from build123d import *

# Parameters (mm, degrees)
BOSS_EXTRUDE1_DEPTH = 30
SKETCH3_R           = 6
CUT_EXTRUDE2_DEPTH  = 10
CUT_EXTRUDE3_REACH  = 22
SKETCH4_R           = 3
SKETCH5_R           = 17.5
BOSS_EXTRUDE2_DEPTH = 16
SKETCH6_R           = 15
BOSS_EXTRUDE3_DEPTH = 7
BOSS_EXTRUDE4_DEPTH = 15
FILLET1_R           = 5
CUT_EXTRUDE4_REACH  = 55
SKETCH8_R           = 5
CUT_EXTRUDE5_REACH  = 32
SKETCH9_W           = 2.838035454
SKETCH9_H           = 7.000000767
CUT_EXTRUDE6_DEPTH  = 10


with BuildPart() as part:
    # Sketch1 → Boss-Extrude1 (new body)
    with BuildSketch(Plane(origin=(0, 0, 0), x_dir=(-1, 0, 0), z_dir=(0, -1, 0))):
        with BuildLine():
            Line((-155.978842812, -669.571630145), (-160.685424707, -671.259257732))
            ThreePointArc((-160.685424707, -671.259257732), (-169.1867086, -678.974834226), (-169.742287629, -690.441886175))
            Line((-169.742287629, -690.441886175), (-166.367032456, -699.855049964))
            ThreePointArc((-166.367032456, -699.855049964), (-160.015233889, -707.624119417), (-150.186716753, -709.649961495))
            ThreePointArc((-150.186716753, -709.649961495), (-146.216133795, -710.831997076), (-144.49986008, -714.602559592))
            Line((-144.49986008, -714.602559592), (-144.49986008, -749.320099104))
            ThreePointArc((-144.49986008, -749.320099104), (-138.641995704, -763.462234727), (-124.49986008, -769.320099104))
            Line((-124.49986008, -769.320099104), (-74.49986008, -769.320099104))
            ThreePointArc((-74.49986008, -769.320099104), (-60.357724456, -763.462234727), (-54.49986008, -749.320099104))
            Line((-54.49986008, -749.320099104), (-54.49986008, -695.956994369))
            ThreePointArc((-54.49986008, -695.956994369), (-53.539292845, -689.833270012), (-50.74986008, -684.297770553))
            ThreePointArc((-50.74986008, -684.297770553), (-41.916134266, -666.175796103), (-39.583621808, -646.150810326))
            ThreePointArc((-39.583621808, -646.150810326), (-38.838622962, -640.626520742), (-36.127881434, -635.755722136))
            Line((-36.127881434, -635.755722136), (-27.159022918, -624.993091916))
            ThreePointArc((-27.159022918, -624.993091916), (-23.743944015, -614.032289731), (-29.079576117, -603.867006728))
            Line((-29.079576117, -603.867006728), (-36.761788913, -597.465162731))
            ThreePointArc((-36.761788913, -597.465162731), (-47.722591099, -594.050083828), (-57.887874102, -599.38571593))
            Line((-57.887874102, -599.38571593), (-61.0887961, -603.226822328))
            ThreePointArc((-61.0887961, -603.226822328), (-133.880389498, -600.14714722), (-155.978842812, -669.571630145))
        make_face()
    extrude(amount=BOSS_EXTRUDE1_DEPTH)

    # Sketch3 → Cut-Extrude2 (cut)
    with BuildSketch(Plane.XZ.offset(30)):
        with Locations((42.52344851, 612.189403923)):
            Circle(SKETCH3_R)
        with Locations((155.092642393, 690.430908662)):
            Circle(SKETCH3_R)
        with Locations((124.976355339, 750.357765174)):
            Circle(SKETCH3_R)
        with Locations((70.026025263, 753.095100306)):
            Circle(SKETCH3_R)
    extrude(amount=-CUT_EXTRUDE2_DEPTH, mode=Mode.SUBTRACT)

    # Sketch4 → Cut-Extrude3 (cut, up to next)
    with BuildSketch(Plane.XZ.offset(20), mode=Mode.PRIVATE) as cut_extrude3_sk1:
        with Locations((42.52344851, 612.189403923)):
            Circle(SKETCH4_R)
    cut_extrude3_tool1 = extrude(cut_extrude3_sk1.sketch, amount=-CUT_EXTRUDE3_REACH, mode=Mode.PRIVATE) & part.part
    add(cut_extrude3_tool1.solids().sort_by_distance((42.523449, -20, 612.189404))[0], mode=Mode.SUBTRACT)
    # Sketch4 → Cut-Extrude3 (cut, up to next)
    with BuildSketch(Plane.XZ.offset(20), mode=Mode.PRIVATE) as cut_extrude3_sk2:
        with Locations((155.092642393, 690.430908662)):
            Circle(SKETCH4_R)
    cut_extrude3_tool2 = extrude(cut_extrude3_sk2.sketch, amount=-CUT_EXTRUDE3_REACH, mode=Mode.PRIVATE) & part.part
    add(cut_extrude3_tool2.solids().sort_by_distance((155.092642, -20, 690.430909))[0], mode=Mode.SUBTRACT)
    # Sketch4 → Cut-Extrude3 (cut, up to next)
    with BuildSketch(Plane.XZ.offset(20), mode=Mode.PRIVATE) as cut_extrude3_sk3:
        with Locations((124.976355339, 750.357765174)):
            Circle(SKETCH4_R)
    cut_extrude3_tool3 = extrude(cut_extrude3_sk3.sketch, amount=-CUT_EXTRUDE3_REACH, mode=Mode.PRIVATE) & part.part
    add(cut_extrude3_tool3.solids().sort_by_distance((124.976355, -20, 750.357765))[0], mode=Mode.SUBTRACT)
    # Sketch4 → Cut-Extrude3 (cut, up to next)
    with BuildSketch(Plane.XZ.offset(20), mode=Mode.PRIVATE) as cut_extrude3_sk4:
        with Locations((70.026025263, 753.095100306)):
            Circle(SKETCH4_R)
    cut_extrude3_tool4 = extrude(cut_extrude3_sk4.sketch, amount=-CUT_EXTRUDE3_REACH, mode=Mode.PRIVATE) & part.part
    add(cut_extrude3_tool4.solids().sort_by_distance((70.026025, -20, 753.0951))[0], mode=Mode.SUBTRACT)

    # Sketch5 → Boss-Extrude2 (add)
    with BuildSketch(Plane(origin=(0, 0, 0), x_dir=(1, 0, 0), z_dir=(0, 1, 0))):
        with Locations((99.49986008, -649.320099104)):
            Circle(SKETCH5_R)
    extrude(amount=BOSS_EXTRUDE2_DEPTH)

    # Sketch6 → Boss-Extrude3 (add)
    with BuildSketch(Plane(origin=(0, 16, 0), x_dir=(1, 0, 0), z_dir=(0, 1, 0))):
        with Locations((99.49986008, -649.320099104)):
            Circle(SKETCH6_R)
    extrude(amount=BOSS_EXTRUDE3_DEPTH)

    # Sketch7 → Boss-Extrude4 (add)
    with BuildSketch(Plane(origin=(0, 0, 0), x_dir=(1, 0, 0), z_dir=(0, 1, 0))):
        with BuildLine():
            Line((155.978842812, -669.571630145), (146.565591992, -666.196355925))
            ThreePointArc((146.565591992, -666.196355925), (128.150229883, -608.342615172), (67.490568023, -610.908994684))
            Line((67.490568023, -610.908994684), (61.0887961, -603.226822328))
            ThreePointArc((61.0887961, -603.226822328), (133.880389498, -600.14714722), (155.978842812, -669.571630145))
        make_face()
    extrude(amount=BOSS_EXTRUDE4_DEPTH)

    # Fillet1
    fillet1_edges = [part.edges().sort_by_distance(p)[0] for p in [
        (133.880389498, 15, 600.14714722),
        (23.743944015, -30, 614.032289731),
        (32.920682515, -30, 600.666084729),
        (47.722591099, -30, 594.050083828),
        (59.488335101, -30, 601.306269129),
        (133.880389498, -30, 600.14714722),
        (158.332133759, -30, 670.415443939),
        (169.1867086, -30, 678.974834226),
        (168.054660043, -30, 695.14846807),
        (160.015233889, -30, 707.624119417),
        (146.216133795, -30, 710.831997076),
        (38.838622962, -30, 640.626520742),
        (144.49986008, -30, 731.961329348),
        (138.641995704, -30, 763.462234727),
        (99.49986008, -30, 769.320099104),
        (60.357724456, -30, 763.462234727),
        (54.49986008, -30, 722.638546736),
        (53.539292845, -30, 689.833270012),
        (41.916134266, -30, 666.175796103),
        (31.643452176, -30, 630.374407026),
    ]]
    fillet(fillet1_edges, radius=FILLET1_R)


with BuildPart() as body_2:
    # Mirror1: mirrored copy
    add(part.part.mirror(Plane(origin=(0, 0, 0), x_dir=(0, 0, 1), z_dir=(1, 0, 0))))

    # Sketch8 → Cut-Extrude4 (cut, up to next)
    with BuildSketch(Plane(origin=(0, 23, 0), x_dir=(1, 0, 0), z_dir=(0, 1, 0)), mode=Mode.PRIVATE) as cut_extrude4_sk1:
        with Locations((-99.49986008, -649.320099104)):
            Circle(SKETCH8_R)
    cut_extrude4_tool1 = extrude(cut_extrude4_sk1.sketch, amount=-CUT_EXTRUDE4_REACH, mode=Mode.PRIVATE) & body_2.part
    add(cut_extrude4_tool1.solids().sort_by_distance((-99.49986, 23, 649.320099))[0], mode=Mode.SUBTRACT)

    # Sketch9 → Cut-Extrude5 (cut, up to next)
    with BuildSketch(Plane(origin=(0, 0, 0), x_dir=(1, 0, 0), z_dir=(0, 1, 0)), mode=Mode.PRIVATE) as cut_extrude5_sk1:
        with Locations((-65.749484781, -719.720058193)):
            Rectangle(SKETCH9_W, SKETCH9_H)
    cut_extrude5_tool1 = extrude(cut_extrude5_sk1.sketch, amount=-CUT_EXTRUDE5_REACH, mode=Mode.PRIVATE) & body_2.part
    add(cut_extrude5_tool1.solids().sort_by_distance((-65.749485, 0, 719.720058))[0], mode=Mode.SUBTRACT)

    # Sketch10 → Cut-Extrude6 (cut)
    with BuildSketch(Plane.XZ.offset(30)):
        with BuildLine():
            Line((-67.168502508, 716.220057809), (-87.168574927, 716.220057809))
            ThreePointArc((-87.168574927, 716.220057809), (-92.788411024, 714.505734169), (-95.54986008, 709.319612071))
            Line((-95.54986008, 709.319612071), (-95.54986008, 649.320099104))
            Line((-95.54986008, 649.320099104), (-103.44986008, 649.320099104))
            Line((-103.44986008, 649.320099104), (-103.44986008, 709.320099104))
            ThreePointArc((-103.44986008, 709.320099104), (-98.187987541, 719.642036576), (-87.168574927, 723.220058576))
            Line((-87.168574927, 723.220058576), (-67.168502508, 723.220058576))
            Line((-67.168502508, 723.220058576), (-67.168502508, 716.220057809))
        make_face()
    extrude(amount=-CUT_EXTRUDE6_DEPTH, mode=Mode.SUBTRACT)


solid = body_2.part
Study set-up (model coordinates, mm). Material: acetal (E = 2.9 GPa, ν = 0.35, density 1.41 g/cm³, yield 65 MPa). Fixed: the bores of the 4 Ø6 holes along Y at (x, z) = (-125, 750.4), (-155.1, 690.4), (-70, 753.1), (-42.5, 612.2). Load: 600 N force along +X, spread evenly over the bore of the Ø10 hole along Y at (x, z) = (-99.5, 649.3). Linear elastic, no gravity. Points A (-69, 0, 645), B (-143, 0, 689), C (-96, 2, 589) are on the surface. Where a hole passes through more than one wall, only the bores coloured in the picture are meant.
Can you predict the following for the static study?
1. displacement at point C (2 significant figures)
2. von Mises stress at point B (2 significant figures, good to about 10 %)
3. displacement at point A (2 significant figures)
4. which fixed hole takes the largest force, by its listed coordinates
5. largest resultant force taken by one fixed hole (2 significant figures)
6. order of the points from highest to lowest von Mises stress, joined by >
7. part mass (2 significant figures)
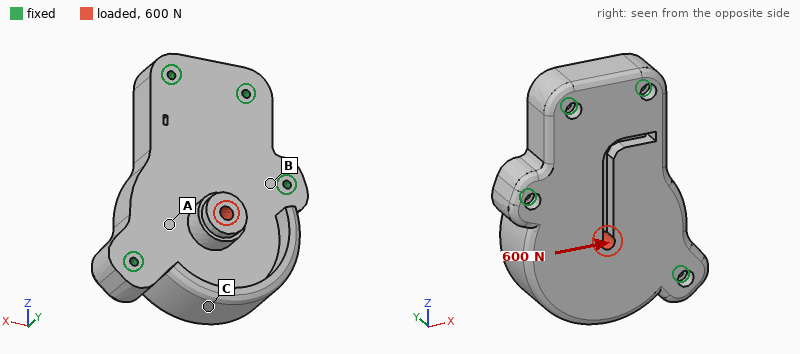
11 µm
0.57 MPa
10 µm
(-42.5, 612.2)
300 N
B > A > C
820 g
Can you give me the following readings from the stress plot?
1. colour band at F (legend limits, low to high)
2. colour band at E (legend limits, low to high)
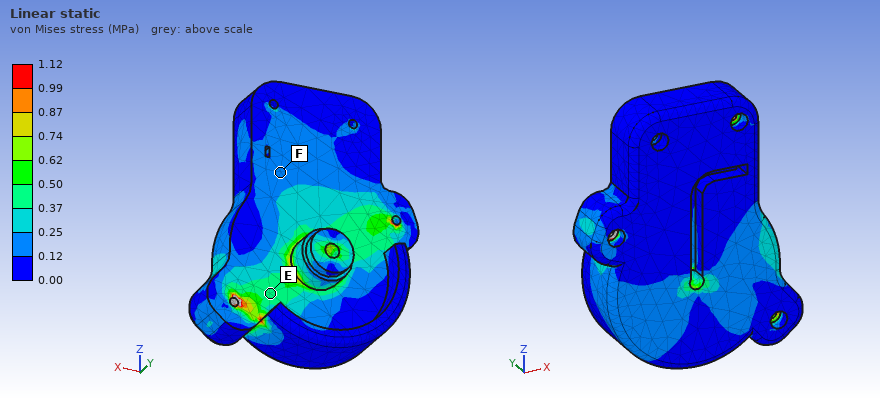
0.12 to 0.25 MPa
0.37 to 0.50 MPa
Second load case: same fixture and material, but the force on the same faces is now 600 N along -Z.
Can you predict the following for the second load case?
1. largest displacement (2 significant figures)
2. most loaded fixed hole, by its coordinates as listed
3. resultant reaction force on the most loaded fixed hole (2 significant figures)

29 µm
(-155.1, 690.4)
180 N
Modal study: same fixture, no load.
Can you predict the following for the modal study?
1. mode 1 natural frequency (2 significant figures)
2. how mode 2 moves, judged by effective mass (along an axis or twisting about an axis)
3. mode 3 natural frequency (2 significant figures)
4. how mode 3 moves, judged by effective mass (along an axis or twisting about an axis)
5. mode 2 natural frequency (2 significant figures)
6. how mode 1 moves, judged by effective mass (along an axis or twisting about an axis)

790 Hz
along Y
2000 Hz
along X
1400 Hz
along Y
